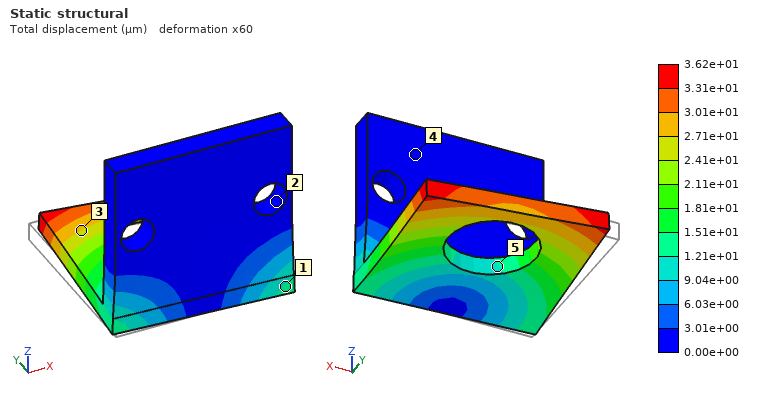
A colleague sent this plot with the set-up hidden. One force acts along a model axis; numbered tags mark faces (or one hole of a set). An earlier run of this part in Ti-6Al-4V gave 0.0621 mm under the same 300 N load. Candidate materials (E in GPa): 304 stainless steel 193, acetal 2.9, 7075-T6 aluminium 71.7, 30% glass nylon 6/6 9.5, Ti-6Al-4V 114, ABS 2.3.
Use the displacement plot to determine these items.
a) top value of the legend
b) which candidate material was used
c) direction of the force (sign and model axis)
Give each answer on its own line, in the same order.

3.62e+01 µm
304 stainless steel
+X
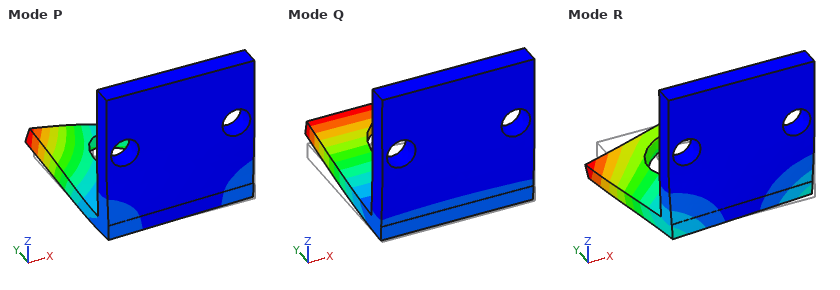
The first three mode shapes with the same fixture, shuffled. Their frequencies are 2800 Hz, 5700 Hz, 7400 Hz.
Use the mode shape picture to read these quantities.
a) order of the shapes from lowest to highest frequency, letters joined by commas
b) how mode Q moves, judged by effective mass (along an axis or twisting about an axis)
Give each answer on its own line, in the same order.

Q, R, P
along Z
